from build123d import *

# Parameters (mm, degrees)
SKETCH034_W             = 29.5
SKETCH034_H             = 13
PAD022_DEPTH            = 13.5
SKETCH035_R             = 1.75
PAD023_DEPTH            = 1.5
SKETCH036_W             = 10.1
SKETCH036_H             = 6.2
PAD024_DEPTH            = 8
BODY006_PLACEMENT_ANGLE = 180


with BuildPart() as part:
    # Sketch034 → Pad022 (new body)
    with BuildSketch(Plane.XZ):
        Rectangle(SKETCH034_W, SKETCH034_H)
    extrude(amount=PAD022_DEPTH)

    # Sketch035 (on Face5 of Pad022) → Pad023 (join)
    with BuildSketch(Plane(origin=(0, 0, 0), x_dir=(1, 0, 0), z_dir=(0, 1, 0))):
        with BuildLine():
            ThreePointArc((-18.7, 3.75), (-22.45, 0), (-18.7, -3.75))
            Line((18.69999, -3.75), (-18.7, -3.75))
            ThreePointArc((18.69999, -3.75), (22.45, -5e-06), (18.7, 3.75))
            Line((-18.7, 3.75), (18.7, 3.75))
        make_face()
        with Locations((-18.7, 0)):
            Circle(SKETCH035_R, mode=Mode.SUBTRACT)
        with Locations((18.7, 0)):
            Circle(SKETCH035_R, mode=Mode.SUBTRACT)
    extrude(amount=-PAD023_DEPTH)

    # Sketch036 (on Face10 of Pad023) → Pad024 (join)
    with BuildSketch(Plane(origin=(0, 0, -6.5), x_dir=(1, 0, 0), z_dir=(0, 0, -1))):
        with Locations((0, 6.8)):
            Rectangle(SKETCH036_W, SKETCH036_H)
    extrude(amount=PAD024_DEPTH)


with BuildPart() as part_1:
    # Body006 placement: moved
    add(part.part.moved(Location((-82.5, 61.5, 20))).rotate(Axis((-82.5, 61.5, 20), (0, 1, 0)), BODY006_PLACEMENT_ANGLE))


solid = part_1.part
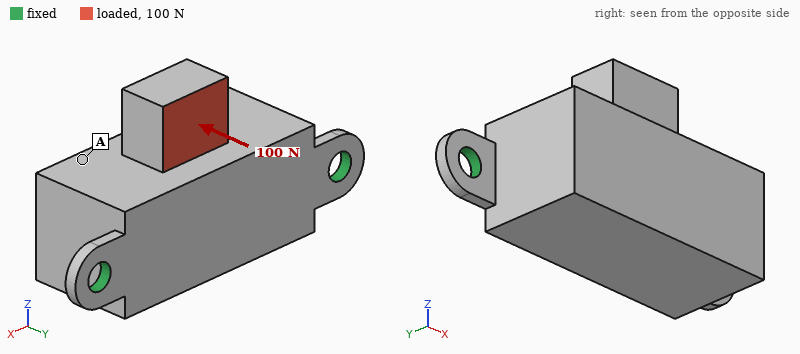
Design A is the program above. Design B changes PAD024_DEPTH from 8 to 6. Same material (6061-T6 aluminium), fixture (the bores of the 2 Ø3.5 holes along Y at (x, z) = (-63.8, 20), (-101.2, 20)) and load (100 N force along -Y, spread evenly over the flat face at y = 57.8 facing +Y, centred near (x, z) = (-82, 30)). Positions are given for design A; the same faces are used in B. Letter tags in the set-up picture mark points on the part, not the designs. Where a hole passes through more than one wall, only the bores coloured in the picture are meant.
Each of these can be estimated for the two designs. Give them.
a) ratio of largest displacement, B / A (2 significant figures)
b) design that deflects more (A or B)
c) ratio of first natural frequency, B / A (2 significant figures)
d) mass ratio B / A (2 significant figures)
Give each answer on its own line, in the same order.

0.82
A
1.0
0.98
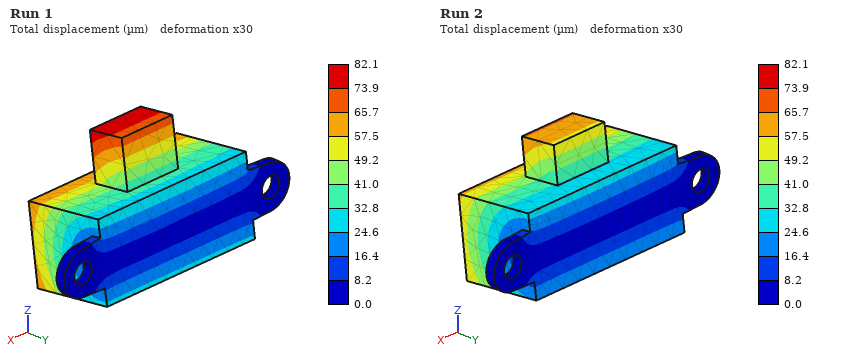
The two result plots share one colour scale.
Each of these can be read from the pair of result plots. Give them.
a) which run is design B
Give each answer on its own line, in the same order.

Run 2
